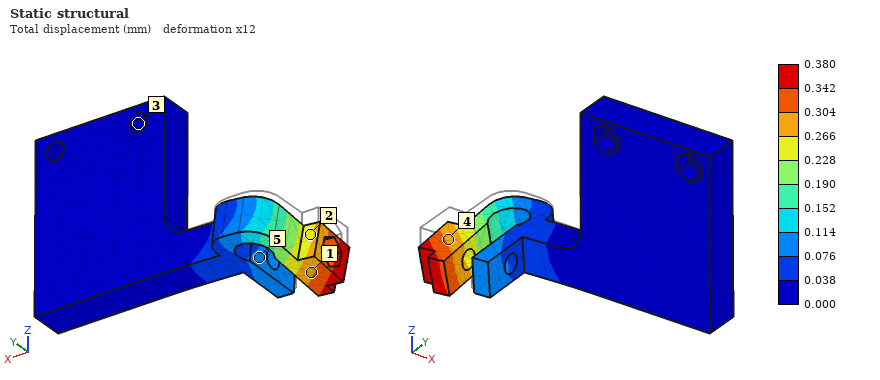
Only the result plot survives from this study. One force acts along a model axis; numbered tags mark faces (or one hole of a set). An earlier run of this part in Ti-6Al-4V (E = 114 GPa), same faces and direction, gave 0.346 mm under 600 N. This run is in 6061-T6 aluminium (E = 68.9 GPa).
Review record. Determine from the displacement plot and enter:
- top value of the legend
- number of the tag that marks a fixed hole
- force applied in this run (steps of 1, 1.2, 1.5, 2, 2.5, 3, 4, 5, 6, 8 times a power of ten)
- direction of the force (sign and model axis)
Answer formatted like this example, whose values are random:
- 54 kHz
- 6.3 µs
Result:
- 0.380 mm
- 3
- 400 N
- -Z
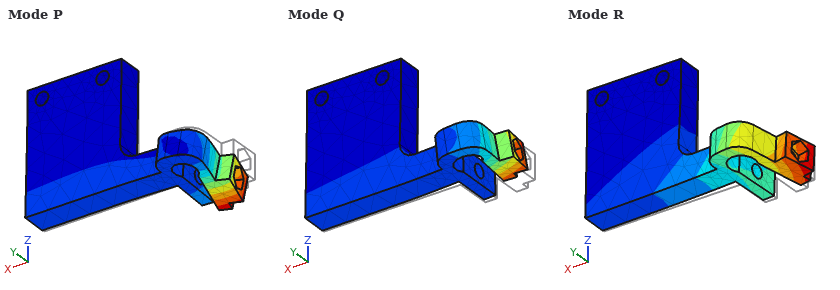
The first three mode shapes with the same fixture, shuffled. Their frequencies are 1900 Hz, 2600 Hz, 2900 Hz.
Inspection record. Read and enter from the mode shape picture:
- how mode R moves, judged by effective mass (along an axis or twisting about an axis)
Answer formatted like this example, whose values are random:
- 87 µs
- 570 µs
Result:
- along Y
